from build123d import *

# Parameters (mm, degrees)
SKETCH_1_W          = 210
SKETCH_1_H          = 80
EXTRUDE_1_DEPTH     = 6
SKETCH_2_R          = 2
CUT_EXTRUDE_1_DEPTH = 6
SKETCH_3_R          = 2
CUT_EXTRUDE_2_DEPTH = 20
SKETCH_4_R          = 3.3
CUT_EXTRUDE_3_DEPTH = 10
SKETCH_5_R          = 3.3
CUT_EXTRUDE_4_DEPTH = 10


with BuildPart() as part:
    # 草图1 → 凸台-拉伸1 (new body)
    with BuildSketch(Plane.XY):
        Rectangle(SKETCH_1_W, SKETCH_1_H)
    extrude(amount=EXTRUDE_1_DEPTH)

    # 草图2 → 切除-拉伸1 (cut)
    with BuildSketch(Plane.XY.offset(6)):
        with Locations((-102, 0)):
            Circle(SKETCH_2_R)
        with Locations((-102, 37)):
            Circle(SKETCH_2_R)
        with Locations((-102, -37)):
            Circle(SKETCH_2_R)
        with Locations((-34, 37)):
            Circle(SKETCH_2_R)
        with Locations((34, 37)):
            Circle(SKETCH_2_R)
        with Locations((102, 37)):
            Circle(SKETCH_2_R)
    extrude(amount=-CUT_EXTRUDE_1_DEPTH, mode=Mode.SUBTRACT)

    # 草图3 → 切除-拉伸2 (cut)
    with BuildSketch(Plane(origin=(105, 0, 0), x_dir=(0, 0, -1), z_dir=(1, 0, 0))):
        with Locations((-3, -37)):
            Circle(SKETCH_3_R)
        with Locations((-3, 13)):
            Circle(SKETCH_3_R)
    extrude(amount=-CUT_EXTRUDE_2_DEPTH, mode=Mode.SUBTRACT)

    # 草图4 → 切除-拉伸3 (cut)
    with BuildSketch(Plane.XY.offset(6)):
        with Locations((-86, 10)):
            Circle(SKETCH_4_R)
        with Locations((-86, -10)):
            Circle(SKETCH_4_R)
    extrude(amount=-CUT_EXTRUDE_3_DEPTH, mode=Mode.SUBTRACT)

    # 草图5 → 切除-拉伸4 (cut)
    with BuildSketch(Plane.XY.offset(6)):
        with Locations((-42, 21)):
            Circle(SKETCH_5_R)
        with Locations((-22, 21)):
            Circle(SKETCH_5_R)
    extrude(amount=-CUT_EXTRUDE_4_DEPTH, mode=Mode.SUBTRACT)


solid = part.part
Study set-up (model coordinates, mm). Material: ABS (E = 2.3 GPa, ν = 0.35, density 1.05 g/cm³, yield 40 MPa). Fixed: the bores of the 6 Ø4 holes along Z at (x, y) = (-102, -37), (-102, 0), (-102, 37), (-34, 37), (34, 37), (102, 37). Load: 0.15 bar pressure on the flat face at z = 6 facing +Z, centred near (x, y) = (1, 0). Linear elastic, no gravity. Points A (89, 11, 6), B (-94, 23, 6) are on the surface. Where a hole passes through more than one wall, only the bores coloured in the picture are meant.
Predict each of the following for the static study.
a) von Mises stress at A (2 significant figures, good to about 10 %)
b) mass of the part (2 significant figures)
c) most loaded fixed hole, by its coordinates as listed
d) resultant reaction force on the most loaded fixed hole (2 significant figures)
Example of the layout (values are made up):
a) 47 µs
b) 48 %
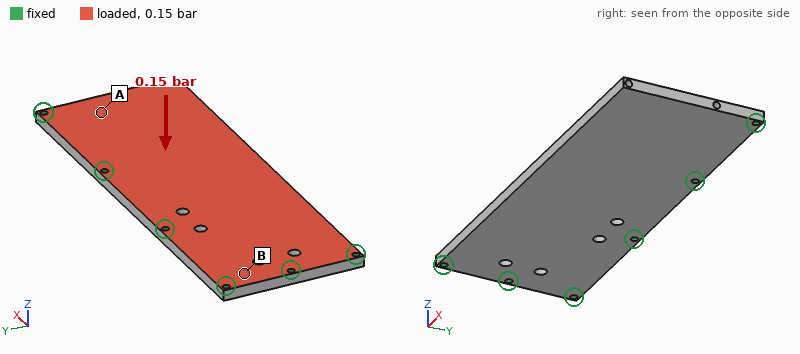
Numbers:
a) 3.0 MPa
b) 100 g
c) (34, 37)
d) 91 N
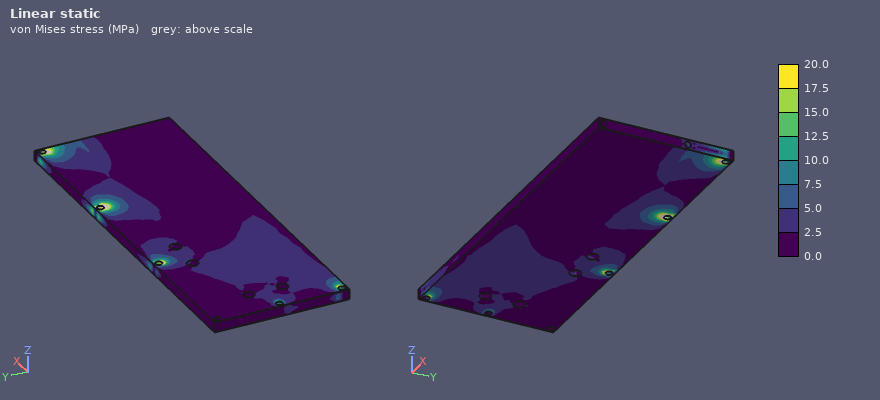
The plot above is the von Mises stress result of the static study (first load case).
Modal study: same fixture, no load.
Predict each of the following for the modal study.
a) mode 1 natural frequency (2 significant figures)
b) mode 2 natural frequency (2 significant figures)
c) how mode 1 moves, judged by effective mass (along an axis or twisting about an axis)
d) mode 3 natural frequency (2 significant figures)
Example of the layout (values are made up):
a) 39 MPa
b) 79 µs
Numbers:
a) 210 Hz
b) 410 Hz
c) along Z
d) 780 Hz
